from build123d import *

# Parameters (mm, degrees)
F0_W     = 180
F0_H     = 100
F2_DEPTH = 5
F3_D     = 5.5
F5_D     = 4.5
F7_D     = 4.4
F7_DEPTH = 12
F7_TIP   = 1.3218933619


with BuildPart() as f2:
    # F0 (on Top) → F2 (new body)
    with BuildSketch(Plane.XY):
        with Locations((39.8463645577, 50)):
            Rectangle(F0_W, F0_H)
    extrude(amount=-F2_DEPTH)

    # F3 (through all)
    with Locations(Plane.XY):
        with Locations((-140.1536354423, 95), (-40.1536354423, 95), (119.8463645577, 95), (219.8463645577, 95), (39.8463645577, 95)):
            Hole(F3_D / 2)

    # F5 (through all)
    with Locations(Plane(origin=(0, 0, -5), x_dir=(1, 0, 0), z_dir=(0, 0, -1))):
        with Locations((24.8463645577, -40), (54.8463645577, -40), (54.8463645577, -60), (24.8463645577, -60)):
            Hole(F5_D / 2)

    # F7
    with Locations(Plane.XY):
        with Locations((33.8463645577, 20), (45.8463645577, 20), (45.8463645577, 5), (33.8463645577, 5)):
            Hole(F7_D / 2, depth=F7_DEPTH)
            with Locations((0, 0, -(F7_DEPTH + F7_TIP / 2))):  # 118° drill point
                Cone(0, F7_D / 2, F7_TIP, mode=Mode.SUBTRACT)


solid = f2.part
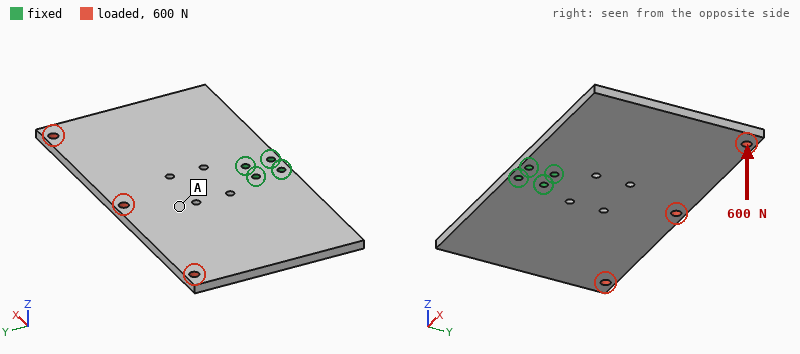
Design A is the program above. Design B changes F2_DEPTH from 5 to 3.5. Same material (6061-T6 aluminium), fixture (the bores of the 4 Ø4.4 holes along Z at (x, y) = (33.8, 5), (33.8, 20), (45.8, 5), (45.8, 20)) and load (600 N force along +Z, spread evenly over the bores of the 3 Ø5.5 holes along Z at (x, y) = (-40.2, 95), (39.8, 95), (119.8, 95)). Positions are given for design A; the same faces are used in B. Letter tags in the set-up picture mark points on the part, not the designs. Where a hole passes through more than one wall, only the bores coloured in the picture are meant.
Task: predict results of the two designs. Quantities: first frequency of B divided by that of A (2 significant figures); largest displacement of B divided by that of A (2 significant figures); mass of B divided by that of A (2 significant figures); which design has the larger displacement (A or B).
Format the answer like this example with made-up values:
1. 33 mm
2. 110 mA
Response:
1. 0.71
2. 2.8
3. 0.70
4. B
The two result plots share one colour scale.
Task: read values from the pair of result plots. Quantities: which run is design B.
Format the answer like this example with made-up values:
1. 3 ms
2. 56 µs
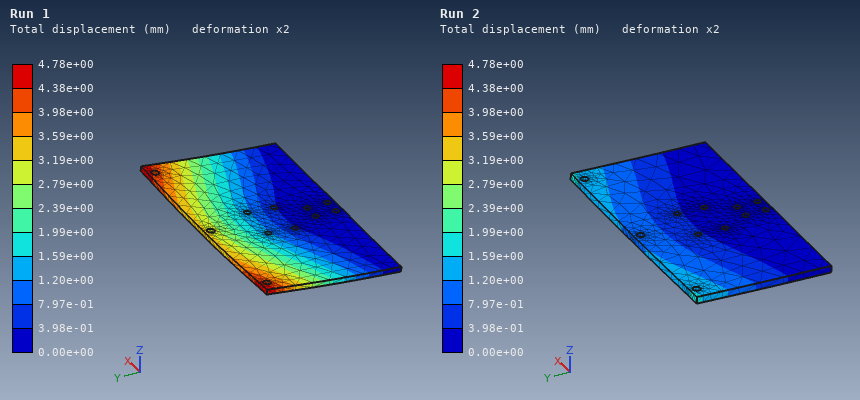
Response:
1. Run 1
